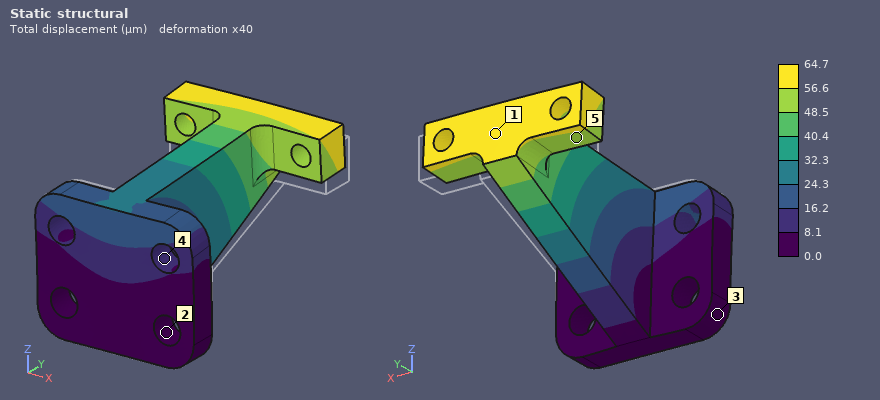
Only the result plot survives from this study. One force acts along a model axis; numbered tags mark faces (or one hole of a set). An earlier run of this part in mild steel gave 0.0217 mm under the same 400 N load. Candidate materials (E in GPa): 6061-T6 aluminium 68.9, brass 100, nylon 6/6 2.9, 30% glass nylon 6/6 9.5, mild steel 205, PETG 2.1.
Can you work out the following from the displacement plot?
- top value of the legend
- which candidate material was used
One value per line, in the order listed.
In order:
64.7 µm
6061-T6 aluminium
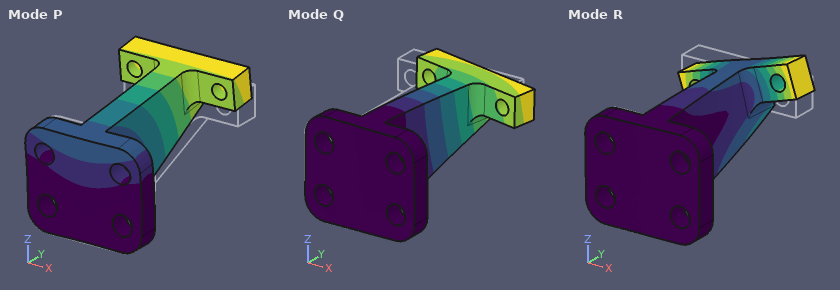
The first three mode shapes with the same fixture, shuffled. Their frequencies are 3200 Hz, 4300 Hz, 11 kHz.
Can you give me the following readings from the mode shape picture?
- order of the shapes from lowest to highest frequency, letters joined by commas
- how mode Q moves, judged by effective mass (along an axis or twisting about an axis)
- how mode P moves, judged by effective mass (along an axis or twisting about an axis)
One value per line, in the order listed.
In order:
Q, P, R
along X
along Z
